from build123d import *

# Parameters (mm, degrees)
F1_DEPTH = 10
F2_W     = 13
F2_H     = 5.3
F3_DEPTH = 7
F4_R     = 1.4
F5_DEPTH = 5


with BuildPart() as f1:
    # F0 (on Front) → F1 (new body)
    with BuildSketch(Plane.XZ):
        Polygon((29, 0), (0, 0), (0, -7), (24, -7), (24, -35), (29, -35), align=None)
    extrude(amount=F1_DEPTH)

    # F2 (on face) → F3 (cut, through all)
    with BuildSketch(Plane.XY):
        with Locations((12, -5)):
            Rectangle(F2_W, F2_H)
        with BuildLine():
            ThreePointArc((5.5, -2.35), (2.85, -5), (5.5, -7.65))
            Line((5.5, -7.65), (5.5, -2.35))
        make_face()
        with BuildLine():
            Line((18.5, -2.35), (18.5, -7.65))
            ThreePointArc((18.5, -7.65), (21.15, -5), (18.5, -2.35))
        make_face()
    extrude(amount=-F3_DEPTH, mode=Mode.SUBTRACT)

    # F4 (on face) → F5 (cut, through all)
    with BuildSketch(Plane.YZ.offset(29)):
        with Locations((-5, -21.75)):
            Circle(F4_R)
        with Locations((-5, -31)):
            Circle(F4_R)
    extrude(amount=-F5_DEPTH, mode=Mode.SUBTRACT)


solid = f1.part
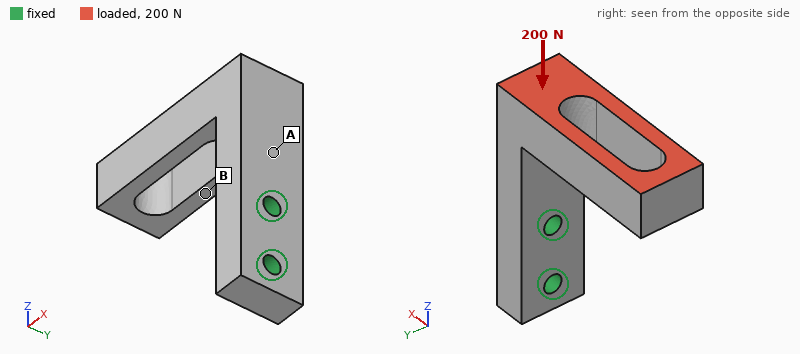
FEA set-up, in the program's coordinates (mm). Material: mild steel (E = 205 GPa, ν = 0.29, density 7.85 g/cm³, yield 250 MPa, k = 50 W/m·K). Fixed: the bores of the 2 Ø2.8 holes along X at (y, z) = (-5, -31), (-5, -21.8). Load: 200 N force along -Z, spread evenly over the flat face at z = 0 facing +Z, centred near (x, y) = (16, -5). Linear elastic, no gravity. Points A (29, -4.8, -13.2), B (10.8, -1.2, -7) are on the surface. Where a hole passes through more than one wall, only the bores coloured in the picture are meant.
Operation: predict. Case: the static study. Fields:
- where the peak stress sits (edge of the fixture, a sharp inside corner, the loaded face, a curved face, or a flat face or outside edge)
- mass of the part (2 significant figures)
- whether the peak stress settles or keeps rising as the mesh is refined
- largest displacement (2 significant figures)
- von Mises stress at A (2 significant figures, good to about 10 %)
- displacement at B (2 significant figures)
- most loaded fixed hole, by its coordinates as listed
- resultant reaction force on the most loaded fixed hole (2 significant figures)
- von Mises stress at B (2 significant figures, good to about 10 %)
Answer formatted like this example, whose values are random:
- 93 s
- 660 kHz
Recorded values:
- edge of the fixture
- 21 g
- keeps rising
- 61 µm
- 47 MPa
- 32 µm
- (-5, -21.8)
- 180 N
- 11 MPa
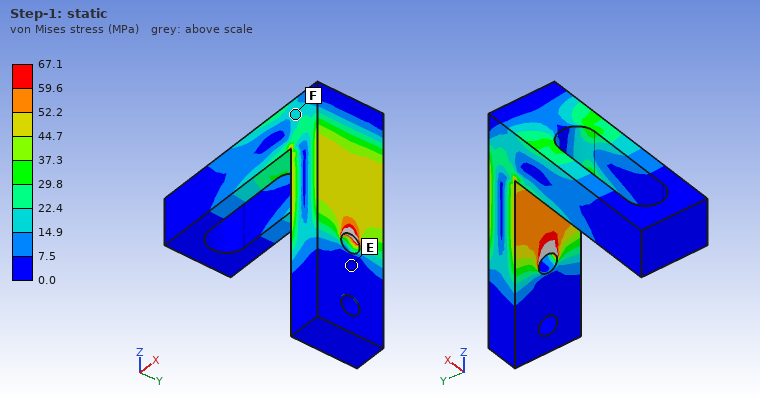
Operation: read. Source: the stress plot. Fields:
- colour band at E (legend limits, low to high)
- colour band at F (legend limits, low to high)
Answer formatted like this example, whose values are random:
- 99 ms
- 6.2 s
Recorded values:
- 0.0 to 7.5 MPa
- 14.9 to 22.4 MPa
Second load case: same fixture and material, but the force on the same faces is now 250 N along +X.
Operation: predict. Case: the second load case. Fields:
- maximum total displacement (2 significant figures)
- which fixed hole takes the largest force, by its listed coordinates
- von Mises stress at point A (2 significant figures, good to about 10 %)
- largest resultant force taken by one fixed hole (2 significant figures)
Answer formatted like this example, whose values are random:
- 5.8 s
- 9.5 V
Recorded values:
- 85 µm
- (-5, -21.8)
- 78 MPa
- 370 N
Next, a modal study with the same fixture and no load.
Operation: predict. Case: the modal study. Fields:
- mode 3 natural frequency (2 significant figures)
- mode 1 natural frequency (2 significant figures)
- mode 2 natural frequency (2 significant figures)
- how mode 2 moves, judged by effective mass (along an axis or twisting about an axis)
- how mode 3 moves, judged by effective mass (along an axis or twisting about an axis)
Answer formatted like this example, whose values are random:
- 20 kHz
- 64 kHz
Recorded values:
- 8900 Hz
- 2900 Hz
- 3200 Hz
- along Y
- along X
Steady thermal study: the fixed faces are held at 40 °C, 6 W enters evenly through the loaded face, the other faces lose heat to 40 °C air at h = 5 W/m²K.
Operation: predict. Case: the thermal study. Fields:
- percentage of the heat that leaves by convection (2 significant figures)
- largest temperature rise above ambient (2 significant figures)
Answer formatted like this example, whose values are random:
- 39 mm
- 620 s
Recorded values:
- 5.1 %
- 68 K
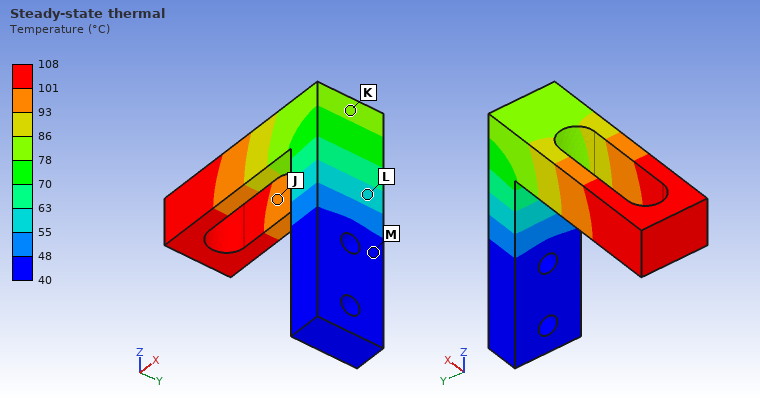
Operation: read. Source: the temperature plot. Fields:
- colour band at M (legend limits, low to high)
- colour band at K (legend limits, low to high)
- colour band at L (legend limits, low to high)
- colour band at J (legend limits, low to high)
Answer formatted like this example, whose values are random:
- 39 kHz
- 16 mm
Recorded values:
- 40 to 48 °C
- 78 to 86 °C
- 55 to 63 °C
- 93 to 101 °C
